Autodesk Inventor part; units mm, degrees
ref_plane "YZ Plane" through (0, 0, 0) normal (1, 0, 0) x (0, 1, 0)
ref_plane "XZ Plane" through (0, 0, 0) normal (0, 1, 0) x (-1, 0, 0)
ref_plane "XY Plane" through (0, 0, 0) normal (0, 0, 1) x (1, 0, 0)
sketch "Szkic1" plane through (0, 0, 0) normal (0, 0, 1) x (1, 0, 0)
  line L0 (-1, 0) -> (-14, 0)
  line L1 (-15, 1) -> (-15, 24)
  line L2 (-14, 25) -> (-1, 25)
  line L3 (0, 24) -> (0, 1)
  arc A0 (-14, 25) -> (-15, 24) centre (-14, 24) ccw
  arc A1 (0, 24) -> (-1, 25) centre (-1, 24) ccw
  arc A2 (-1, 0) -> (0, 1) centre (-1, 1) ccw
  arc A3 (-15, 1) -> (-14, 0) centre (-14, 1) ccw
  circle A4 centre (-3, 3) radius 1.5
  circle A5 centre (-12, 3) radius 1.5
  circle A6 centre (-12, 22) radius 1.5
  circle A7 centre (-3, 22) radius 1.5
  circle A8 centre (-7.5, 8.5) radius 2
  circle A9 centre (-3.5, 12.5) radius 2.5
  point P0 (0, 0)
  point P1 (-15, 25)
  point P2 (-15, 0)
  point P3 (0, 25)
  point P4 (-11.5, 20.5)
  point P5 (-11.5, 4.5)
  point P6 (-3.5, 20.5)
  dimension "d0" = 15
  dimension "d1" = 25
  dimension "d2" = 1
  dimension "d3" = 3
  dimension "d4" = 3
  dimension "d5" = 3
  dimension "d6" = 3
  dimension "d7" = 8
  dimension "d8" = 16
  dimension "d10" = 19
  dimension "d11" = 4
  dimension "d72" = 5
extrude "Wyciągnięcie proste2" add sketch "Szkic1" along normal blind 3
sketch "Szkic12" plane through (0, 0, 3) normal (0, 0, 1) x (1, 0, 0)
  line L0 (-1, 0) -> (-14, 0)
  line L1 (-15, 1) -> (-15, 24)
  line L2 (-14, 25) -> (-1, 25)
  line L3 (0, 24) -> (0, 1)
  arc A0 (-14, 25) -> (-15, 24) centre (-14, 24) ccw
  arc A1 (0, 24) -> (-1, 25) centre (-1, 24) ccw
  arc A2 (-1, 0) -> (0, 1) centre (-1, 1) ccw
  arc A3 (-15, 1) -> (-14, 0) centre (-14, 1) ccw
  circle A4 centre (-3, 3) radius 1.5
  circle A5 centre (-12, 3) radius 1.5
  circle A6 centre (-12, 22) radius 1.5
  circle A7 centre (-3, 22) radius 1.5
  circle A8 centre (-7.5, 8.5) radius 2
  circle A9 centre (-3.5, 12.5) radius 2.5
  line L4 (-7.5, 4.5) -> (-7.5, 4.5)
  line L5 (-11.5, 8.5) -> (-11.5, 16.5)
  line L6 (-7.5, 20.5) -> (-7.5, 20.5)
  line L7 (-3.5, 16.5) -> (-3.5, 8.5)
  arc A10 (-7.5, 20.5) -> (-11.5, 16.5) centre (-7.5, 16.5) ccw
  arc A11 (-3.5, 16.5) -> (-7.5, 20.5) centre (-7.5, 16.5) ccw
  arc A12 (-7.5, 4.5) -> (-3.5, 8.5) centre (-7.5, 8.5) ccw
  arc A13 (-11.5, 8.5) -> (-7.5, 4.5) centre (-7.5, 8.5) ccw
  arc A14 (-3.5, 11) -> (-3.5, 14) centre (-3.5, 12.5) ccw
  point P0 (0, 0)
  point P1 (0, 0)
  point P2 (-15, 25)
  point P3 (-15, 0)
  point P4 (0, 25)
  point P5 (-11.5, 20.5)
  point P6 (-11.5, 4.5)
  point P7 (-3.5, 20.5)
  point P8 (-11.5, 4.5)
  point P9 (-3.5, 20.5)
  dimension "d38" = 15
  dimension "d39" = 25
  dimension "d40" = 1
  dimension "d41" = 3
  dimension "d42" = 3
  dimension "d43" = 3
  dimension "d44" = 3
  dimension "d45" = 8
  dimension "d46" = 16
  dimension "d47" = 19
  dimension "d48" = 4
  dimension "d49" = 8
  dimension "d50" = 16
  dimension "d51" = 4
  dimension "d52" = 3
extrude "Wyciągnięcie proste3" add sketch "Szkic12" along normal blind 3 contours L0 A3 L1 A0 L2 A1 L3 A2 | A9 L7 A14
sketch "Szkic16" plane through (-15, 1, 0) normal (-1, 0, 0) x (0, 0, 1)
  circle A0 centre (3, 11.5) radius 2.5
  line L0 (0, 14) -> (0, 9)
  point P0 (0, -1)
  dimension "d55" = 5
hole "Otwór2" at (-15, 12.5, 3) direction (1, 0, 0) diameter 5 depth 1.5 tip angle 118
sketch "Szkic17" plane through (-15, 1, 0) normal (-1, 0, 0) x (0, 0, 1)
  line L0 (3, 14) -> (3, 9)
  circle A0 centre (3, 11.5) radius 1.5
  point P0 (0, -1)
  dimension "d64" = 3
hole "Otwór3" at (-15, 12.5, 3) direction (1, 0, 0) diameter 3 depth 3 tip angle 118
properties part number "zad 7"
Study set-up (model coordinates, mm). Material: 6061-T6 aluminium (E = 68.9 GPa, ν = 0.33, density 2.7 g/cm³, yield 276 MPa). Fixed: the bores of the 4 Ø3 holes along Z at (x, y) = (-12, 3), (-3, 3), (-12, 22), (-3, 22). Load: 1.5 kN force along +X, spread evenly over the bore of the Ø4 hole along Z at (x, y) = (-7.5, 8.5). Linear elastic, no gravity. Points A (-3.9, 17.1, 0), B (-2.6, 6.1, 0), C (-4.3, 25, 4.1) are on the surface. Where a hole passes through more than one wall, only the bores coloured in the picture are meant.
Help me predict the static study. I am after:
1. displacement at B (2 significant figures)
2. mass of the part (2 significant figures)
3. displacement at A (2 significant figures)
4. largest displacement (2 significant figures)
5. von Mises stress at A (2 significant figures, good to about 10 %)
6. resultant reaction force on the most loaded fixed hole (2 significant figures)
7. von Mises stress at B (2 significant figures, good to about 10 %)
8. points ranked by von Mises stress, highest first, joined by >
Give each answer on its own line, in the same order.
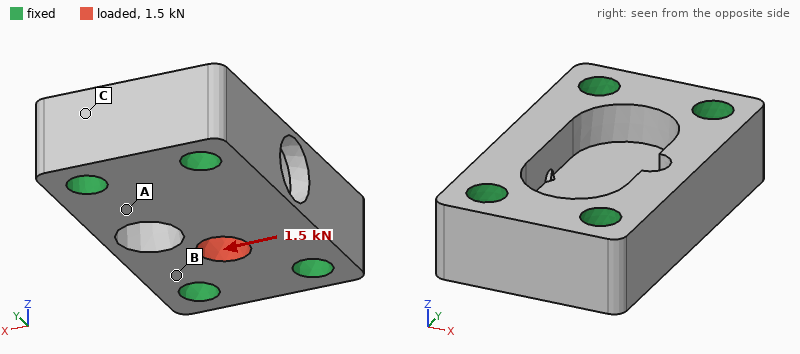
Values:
2.2 µm
4.3 g
1.4 µm
8.3 µm
21 MPa
640 N
40 MPa
B > A > C
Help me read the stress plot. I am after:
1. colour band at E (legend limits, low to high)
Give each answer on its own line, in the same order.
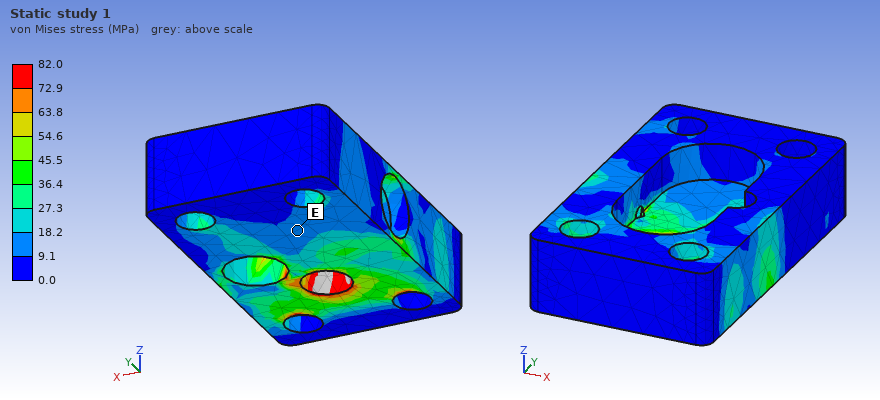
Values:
9.1 to 18.2 MPa
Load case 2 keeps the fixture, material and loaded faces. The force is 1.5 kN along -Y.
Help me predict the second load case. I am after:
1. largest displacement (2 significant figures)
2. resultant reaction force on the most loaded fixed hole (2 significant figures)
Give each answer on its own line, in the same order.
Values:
4.9 µm
590 N
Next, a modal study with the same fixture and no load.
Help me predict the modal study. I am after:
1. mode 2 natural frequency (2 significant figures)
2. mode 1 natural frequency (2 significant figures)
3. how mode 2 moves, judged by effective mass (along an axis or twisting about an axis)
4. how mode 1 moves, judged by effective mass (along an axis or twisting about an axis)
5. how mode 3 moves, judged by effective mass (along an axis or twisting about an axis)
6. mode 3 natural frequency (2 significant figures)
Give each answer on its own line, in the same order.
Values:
72 kHz
66 kHz
along X
along Z
along X
79 kHz
